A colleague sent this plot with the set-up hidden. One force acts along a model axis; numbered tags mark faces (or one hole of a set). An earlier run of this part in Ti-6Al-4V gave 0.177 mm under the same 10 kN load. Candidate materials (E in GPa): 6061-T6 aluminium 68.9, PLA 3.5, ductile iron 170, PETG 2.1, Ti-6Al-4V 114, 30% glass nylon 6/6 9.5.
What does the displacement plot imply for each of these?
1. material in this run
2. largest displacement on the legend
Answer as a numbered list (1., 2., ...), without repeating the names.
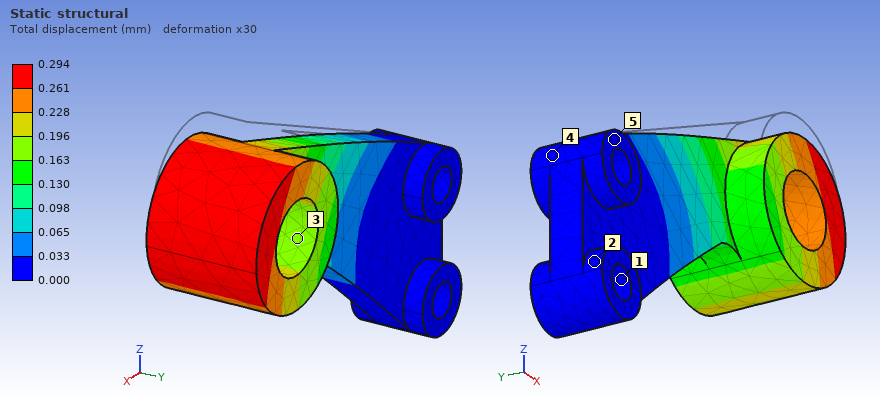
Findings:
1. 6061-T6 aluminium
2. 0.294 mm
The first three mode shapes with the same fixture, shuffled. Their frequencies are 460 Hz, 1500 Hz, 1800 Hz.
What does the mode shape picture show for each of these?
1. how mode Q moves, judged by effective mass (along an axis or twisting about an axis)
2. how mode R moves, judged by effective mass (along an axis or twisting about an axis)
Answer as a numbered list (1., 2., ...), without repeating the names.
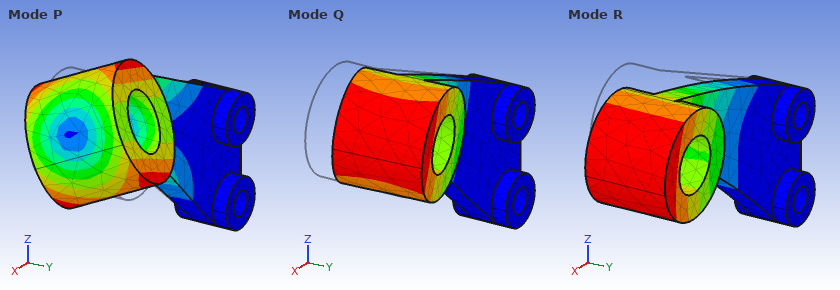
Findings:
1. along Y
2. along Z
